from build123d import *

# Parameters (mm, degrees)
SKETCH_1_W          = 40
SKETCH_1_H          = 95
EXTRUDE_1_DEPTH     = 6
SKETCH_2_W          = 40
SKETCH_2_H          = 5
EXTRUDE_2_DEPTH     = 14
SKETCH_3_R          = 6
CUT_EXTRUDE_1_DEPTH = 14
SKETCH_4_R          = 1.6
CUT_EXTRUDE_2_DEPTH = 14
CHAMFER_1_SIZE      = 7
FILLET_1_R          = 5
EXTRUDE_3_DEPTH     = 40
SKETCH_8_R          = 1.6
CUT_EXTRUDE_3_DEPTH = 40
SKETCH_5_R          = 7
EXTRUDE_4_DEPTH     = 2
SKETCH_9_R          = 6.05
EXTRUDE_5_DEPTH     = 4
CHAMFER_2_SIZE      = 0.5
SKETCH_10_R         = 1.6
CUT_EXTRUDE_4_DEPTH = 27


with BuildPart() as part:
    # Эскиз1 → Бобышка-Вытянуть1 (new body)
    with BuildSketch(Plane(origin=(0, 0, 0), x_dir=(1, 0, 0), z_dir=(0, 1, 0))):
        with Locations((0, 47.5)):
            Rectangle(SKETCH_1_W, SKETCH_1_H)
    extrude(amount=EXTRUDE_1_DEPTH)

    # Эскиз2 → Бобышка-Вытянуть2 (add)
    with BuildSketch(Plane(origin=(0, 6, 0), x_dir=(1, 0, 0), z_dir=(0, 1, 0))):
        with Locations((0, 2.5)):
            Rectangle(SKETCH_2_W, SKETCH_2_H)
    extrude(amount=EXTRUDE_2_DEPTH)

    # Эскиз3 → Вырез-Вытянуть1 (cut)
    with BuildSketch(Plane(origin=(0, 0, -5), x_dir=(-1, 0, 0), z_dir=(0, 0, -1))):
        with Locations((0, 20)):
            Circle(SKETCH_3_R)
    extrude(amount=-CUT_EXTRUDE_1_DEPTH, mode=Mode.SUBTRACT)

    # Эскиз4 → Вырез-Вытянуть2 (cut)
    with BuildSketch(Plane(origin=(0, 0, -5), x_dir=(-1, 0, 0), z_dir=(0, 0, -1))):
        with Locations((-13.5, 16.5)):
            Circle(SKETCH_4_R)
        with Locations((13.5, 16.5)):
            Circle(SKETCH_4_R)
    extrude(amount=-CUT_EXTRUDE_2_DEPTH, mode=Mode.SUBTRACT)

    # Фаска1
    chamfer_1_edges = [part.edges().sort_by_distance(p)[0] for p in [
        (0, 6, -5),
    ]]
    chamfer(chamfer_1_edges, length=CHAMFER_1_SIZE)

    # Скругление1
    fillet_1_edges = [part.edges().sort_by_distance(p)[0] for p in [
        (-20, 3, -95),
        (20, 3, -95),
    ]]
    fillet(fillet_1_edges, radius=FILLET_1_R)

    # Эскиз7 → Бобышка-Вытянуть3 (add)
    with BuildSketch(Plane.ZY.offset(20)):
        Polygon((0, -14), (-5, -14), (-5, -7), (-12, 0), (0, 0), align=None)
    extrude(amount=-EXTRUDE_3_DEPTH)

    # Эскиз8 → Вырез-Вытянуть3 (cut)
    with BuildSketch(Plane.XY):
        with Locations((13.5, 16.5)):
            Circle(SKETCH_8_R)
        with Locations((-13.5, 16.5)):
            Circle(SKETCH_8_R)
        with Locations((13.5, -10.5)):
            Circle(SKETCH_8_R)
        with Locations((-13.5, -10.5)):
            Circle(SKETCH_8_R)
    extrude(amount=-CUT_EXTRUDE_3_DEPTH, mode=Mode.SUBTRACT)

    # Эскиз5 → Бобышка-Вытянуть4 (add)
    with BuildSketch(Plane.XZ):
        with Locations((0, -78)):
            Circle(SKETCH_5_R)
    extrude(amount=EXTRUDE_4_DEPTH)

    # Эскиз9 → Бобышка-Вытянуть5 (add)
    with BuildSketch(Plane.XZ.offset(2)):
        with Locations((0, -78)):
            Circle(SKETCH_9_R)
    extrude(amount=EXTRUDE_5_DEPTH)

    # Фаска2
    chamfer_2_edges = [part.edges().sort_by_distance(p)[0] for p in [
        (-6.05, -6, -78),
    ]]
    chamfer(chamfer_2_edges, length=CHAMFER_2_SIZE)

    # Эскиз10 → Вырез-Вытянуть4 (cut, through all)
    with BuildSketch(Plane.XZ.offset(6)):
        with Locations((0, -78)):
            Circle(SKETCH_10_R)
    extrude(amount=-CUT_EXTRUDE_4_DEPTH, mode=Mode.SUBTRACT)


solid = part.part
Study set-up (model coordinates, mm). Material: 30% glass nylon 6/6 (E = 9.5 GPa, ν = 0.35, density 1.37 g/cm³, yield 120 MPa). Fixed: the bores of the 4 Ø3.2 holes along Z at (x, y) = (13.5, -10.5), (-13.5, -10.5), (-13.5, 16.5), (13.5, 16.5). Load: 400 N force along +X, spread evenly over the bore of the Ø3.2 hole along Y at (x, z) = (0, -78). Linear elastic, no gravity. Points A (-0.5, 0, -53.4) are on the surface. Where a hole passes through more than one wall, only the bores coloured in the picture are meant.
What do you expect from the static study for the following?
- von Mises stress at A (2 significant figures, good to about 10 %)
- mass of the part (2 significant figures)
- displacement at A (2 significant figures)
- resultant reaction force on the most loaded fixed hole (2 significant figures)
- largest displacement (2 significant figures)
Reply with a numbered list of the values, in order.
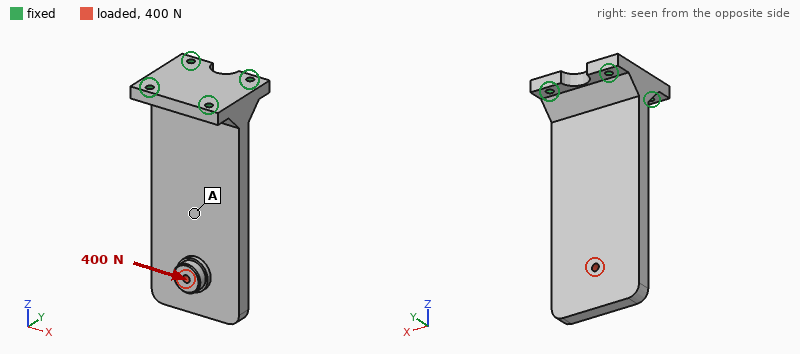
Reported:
1. 8.8 MPa
2. 42 g
3. 0.24 mm
4. 610 N
5. 0.51 mm
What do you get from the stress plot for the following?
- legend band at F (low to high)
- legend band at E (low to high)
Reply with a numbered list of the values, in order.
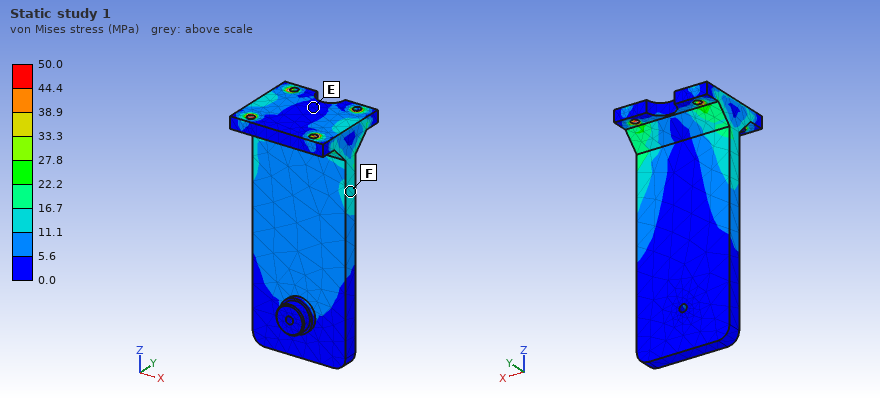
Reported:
1. 11.1 to 16.7 MPa
2. 0.0 to 5.6 MPa
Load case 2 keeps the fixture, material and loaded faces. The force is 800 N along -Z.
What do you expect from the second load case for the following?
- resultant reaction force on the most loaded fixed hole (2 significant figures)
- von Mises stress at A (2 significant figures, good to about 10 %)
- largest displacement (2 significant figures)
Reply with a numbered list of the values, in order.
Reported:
1. 270 N
2. 13 MPa
3. 1.2 mm
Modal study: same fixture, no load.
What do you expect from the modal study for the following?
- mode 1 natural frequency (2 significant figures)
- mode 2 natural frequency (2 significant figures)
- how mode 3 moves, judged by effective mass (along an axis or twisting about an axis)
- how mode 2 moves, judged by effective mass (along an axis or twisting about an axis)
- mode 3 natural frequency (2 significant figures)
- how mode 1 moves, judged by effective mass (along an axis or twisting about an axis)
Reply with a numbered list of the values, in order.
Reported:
1. 340 Hz
2. 1300 Hz
3. twisting about Z
4. along X
5. 1500 Hz
6. along Y
